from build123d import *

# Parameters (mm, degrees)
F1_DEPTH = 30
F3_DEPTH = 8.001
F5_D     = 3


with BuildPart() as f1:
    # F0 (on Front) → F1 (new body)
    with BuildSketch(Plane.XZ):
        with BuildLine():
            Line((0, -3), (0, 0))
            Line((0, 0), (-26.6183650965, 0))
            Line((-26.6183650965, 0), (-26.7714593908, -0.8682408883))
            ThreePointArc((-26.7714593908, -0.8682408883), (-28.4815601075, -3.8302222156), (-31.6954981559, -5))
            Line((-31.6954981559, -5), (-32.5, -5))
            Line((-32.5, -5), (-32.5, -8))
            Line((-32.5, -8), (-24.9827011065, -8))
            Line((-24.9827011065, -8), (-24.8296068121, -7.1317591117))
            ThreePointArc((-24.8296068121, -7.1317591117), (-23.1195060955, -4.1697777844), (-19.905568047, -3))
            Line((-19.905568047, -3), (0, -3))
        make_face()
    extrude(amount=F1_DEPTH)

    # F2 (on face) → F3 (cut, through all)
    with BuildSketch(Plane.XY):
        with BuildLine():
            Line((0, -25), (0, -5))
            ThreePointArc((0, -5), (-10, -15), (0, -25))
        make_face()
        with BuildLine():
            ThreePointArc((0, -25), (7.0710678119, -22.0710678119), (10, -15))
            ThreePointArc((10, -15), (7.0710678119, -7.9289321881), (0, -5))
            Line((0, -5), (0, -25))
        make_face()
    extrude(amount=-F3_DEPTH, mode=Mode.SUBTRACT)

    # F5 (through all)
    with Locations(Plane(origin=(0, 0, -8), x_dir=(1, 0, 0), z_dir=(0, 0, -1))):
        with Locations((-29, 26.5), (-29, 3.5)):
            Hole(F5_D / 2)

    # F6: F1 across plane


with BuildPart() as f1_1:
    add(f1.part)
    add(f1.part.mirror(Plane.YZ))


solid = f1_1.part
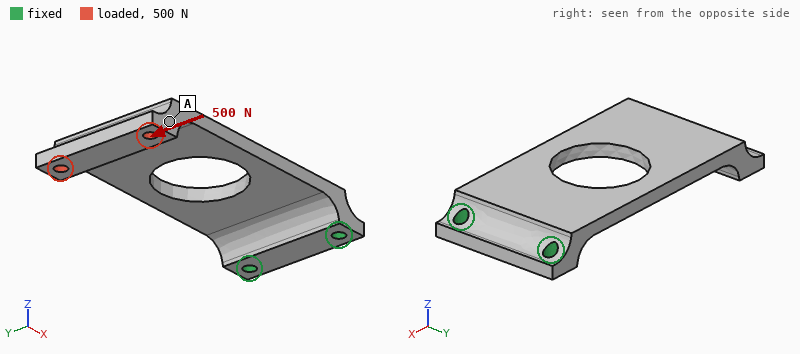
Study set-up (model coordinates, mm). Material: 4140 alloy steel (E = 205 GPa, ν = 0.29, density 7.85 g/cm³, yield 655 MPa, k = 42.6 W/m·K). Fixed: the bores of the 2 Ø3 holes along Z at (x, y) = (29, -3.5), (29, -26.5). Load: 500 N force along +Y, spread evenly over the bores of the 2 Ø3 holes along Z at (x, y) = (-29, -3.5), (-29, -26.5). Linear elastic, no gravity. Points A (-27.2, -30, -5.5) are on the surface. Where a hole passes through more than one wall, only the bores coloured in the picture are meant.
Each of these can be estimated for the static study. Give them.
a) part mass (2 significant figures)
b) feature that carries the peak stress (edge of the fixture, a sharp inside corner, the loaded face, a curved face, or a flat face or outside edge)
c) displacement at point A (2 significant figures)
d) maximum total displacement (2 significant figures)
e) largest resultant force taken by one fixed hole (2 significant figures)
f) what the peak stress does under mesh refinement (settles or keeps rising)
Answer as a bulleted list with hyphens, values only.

- 47 g
- edge of the fixture
- 0.13 mm
- 0.15 mm
- 1.2 kN
- keeps rising
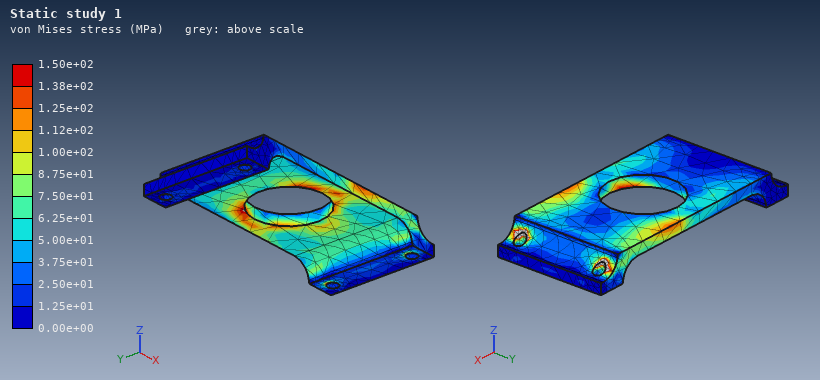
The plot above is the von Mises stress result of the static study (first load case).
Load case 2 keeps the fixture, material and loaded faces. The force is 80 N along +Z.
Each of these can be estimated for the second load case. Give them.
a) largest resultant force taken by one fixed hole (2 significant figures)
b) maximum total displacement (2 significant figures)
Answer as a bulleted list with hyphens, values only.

- 58 N
- 0.52 mm
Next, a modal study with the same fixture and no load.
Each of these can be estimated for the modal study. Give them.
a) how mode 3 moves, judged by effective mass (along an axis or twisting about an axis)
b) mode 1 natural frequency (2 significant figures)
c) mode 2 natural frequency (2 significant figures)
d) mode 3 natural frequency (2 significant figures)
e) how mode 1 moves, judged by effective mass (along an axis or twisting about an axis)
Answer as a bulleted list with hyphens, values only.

- along Y
- 550 Hz
- 2200 Hz
- 3800 Hz
- along Z
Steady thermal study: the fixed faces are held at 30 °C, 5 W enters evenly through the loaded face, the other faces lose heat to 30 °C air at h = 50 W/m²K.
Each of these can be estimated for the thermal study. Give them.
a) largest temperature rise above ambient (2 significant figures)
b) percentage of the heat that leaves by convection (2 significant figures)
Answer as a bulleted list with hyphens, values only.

- 45 K
- 78 %
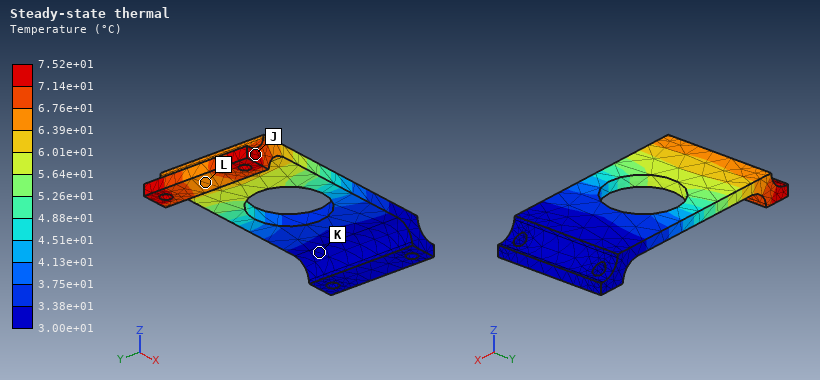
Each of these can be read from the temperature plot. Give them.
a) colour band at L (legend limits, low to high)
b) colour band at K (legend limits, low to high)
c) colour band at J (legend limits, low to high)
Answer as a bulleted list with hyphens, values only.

- 6.39e+01 to 6.76e+01 °C
- 3.00e+01 to 3.38e+01 °C
- 7.14e+01 to 7.52e+01 °C
